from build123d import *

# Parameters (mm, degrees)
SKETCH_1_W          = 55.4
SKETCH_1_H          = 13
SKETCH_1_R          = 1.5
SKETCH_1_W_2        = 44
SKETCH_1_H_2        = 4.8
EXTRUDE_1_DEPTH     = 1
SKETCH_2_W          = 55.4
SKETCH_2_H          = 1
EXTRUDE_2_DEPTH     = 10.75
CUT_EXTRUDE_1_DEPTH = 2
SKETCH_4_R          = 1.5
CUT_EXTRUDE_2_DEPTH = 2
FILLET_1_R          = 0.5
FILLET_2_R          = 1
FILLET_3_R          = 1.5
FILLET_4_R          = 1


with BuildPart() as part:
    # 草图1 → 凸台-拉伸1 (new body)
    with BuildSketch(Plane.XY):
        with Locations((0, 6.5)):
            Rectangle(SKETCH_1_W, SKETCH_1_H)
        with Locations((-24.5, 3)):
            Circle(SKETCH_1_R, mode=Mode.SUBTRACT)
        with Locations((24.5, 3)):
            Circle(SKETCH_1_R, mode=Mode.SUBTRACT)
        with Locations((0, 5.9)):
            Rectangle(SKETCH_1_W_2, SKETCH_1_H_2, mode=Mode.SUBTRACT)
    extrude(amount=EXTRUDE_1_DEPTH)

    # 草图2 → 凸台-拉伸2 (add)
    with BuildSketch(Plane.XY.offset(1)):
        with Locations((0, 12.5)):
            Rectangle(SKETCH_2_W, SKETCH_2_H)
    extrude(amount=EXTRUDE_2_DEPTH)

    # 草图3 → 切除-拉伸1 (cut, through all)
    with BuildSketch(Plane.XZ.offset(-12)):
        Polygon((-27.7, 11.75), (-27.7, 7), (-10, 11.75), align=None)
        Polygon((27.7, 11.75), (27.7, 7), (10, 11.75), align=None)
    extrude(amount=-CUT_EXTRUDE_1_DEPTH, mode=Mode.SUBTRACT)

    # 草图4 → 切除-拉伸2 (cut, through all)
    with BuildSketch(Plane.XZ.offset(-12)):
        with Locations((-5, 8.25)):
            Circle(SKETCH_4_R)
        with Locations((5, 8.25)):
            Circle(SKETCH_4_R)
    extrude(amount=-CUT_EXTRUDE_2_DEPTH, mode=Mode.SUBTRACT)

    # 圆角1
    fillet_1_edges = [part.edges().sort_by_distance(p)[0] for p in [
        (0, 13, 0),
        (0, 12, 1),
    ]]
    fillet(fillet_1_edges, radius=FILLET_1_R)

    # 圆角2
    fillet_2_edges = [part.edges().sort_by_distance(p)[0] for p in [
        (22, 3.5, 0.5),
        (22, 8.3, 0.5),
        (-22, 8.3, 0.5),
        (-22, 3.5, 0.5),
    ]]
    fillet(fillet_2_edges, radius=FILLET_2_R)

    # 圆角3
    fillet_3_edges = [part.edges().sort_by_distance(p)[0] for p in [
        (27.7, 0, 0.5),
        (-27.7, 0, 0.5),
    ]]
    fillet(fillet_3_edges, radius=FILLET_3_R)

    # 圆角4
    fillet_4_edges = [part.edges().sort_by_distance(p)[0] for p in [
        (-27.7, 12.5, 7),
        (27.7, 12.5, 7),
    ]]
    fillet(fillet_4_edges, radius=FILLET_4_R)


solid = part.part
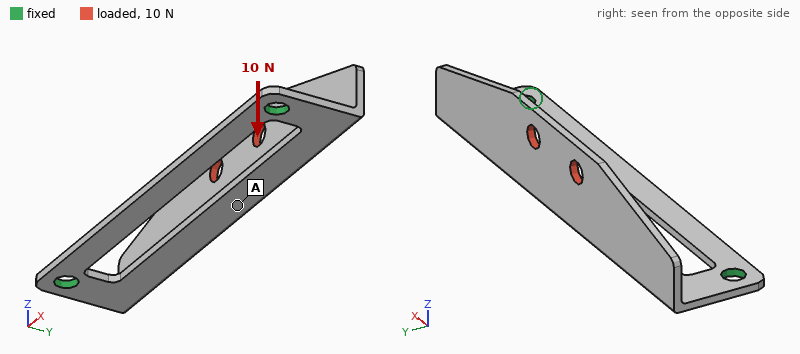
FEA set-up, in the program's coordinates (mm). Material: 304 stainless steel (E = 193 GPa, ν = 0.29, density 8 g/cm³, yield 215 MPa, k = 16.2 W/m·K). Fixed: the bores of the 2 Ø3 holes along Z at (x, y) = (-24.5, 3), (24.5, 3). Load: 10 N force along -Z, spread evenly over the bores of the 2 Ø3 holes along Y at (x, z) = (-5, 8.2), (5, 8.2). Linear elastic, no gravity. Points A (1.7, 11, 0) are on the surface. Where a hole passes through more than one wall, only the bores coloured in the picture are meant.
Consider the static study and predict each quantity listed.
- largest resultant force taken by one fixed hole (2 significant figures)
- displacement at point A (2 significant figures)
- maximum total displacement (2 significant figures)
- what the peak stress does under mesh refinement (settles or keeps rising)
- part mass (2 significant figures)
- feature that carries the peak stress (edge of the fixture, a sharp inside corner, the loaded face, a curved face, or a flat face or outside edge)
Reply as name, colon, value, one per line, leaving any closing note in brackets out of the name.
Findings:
largest resultant force taken by one fixed hole: 5.0 N
displacement at point A: 8.2 µm
maximum total displacement: 23 µm
what the peak stress does under mesh refinement: keeps rising
part mass: 7.9 g
feature that carries the peak stress: edge of the fixture
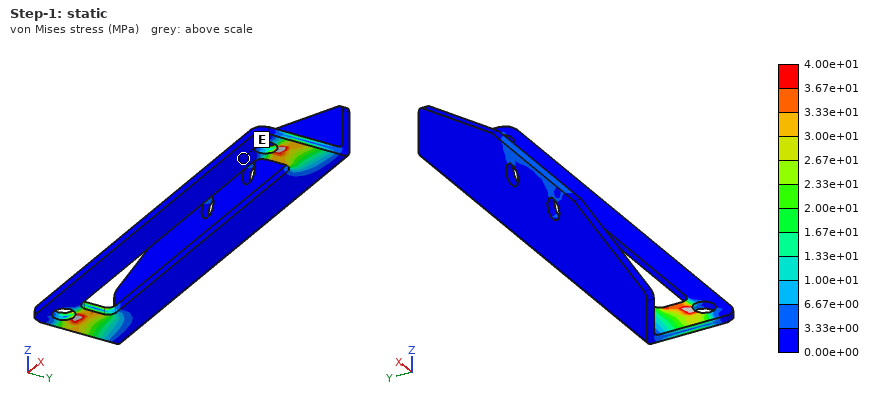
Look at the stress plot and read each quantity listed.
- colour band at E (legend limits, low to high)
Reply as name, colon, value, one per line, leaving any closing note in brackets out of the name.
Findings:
colour band at E: 0.00e+00 to 3.33e+00 MPa
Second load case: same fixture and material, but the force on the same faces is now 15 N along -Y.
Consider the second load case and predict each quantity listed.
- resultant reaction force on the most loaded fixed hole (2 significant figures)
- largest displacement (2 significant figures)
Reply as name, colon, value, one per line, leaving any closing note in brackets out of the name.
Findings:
resultant reaction force on the most loaded fixed hole: 13 N
largest displacement: 85 µm
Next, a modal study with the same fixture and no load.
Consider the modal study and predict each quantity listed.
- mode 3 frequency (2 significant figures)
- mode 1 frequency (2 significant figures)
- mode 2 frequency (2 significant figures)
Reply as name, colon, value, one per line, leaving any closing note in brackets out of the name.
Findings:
mode 3 frequency: 3700 Hz
mode 1 frequency: 1500 Hz
mode 2 frequency: 2400 Hz
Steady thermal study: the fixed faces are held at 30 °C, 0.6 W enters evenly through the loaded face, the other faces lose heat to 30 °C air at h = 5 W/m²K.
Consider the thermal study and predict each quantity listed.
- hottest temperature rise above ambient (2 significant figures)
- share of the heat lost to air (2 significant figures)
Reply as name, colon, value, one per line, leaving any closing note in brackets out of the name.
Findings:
hottest temperature rise above ambient: 41 K
share of the heat lost to air: 35 %
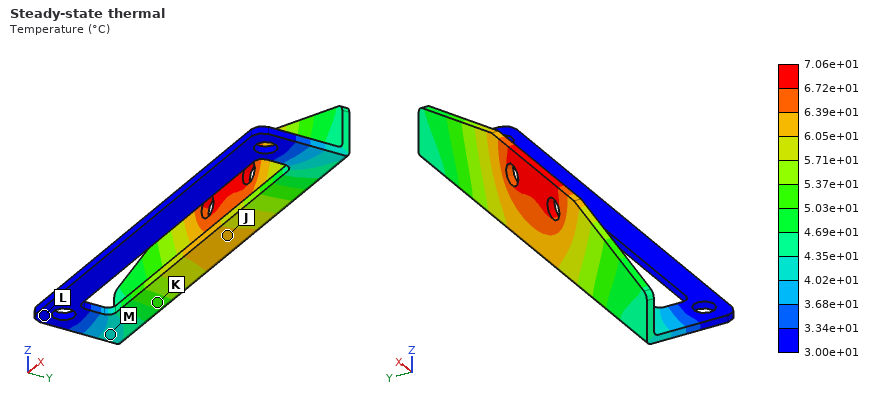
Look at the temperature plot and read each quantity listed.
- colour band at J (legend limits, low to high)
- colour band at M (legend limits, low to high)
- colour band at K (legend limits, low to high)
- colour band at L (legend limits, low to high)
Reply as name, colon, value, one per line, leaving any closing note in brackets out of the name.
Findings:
colour band at J: 6.05e+01 to 6.39e+01 °C
colour band at M: 4.02e+01 to 4.35e+01 °C
colour band at K: 5.03e+01 to 5.37e+01 °C
colour band at L: 3.00e+01 to 3.34e+01 °C
